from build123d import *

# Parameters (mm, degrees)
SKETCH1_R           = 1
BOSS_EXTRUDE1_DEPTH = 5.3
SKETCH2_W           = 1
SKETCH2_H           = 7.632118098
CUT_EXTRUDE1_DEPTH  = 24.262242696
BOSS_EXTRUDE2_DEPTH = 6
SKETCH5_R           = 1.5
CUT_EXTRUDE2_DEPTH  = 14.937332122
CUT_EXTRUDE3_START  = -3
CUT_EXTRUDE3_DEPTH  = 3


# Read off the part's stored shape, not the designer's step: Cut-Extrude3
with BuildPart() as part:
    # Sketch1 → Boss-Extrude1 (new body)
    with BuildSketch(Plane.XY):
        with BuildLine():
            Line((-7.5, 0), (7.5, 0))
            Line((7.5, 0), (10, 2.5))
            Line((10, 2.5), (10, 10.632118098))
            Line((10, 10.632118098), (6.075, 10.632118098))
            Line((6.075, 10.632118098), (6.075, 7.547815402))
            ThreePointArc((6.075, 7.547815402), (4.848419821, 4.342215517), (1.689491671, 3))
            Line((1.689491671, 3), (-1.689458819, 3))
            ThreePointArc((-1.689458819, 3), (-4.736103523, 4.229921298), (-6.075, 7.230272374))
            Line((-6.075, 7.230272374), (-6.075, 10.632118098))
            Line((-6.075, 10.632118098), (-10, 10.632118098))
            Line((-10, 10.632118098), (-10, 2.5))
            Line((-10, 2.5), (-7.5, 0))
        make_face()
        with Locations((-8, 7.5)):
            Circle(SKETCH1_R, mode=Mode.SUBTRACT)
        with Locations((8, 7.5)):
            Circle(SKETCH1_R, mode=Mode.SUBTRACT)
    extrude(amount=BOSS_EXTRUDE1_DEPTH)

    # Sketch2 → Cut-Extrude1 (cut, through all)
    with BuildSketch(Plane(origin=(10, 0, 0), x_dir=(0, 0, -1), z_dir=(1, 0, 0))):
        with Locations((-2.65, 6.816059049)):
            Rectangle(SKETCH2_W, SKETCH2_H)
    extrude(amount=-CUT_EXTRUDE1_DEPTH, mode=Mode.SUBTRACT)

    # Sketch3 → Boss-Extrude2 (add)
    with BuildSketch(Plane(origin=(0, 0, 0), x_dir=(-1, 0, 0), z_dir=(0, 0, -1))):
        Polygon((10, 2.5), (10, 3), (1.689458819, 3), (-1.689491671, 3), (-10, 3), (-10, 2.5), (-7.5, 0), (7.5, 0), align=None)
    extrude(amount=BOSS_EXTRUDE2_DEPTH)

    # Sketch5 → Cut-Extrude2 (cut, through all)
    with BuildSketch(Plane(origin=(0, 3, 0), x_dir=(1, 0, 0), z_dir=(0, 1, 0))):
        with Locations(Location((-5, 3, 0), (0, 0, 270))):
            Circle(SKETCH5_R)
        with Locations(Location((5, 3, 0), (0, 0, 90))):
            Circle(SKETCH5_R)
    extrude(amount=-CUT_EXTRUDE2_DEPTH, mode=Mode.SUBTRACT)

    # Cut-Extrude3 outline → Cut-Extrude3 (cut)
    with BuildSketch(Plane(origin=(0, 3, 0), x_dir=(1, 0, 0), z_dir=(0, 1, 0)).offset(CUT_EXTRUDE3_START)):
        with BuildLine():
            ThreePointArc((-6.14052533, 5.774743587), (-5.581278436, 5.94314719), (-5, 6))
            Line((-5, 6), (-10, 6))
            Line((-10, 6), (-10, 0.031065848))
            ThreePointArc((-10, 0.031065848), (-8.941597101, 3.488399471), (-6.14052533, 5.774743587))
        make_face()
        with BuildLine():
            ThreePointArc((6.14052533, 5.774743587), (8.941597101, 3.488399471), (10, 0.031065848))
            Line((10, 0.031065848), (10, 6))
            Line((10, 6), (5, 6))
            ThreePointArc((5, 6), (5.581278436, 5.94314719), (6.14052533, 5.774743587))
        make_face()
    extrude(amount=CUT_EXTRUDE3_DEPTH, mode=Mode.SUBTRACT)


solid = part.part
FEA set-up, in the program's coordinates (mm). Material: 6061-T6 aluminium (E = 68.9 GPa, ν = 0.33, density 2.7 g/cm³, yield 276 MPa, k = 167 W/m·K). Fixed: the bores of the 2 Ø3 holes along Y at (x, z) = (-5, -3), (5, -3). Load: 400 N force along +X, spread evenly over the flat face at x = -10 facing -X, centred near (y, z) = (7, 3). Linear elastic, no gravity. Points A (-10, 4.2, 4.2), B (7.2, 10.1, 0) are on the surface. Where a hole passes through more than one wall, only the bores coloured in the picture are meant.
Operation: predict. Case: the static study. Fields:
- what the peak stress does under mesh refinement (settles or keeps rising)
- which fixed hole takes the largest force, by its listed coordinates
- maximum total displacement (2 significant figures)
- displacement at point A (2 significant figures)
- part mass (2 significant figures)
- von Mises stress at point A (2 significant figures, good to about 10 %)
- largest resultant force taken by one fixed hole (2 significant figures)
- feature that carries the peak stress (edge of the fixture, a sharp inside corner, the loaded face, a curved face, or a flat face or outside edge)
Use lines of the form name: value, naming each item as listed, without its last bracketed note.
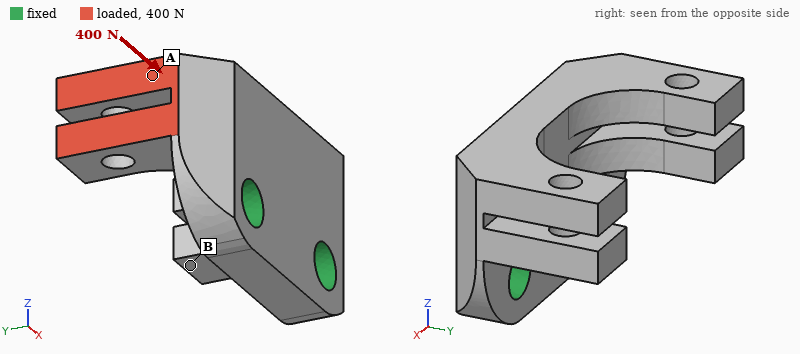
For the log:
what the peak stress does under mesh refinement: keeps rising
which fixed hole takes the largest force, by its listed coordinates: (-5, -3)
maximum total displacement: 65 µm
displacement at point A: 31 µm
part mass: 2.2 g
von Mises stress at point A: 54 MPa
largest resultant force taken by one fixed hole: 300 N
feature that carries the peak stress: edge of the fixture
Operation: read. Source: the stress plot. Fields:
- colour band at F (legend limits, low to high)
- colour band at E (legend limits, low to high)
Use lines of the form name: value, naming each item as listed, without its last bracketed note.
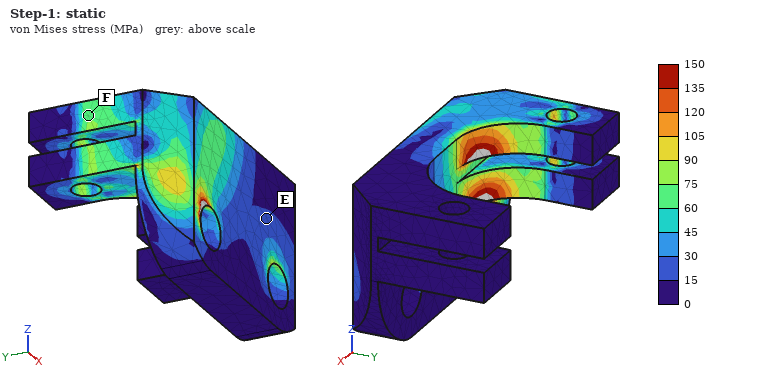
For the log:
colour band at F: 60 to 75 MPa
colour band at E: 15 to 30 MPa
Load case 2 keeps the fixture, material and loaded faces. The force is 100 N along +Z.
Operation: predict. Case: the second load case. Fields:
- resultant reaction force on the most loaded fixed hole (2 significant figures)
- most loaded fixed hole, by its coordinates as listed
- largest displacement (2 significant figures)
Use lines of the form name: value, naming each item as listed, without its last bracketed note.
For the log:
resultant reaction force on the most loaded fixed hole: 130 N
most loaded fixed hole, by its coordinates as listed: (-5, -3)
largest displacement: 40 µm
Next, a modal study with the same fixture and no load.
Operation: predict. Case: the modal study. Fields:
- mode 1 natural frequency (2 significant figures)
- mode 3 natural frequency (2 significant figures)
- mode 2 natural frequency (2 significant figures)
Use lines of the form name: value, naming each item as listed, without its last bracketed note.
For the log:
mode 1 natural frequency: 17 kHz
mode 3 natural frequency: 24 kHz
mode 2 natural frequency: 18 kHz
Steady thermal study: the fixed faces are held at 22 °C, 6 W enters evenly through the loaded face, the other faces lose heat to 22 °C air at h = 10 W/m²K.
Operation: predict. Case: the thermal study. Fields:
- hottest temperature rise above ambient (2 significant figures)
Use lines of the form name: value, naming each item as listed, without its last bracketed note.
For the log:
hottest temperature rise above ambient: 18 K
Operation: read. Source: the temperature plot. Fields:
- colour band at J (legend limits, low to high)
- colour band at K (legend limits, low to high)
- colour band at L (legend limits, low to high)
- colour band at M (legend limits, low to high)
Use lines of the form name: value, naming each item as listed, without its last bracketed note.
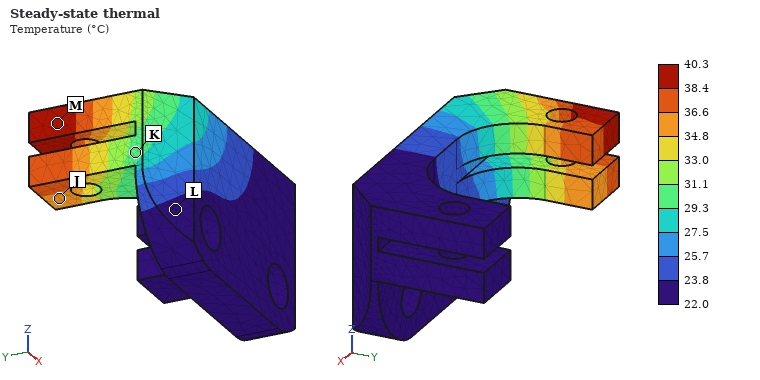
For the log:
colour band at J: 34.8 to 36.6 °C
colour band at K: 29.3 to 31.1 °C
colour band at L: 22.0 to 23.8 °C
colour band at M: 38.4 to 40.3 °C
